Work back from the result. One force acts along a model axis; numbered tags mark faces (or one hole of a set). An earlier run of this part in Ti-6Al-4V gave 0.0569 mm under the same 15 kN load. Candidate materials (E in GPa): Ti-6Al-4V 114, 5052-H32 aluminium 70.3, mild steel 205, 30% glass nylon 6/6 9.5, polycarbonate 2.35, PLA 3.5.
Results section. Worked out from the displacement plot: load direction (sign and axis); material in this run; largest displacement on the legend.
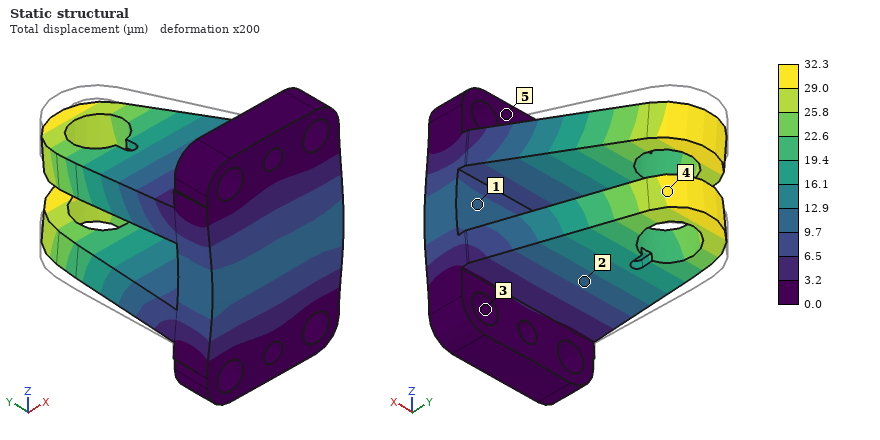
-Y
mild steel
32.3 µm
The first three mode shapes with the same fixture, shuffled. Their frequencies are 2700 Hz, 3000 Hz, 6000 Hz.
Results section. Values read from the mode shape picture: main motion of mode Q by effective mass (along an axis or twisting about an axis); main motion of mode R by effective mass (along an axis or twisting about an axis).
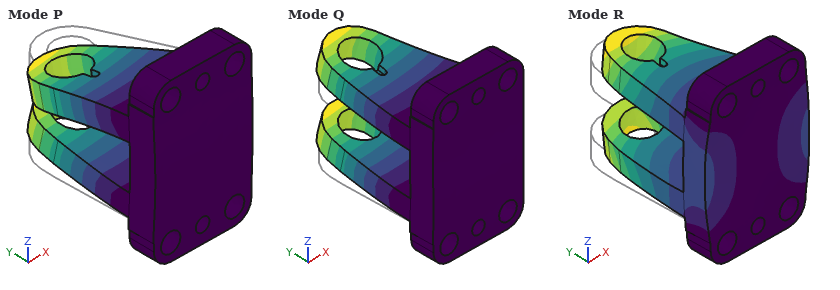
along Z
along X
